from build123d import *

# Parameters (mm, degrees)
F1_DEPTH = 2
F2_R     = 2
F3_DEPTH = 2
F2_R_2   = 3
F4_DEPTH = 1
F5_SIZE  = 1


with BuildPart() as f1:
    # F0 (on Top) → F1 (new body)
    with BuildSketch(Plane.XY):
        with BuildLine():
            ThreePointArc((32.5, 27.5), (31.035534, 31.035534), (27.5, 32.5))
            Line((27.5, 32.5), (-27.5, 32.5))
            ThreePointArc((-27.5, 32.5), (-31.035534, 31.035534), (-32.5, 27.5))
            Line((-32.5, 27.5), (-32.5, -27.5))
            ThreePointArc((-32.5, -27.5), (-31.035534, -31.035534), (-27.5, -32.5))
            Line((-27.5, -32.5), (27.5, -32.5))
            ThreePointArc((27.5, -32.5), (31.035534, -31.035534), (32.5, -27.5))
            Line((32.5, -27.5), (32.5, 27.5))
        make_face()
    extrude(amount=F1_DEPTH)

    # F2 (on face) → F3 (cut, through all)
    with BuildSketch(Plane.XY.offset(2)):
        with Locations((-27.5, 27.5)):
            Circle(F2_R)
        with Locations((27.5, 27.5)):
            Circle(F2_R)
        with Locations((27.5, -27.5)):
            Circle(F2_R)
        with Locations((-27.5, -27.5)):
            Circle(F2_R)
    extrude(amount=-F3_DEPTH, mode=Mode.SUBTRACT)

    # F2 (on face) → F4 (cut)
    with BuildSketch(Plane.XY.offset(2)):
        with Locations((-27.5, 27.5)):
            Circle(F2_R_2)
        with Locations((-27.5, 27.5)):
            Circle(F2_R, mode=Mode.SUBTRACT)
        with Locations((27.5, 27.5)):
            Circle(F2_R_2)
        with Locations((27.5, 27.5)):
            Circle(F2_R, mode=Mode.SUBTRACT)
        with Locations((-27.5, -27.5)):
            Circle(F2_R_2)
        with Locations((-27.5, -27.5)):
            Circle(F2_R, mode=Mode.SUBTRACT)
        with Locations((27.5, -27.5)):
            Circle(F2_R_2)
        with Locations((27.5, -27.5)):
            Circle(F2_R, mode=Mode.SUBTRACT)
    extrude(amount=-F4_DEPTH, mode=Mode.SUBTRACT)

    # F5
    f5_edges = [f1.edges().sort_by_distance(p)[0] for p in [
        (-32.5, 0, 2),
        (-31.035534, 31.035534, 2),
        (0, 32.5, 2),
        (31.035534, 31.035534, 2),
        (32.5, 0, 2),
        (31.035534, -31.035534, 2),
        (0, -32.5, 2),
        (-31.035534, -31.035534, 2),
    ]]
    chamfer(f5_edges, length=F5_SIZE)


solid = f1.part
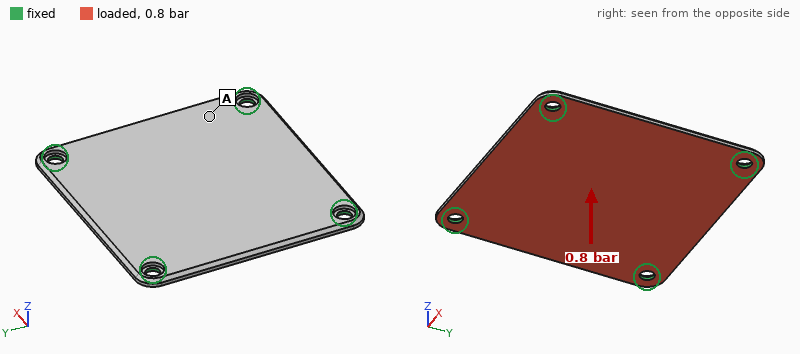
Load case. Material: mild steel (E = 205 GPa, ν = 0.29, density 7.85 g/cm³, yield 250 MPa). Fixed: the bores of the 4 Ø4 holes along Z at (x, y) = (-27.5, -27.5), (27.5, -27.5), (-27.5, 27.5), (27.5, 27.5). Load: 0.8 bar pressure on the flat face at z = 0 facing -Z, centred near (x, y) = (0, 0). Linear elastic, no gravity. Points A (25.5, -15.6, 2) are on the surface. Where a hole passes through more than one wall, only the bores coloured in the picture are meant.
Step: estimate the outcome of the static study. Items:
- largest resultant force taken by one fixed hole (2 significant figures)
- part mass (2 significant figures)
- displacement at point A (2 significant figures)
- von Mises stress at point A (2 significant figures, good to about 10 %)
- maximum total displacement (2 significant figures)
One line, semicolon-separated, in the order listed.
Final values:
180 N; 64 g; 15 µm; 13 MPa; 44 µm
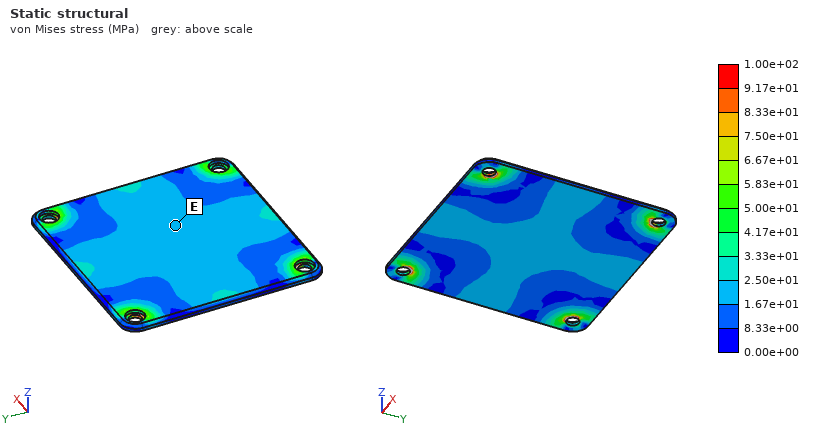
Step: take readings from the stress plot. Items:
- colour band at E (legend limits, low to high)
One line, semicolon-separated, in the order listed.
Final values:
1.67e+01 to 2.50e+01 MPa
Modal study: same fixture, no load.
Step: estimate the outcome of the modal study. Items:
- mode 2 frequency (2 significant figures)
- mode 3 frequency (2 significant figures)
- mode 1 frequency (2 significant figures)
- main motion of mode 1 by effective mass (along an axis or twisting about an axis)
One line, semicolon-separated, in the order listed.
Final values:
3600 Hz; 3600 Hz; 2100 Hz; along Z
